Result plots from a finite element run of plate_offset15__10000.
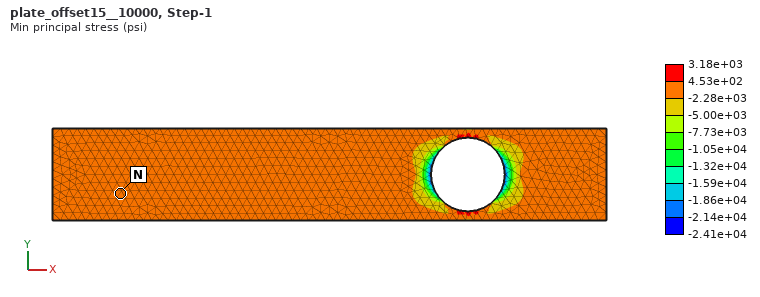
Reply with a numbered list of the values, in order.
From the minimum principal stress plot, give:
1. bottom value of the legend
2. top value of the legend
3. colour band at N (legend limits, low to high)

1. -2.41e+04 psi
2. 3.18e+03 psi
3. -2.28e+03 to 4.53e+02 psi
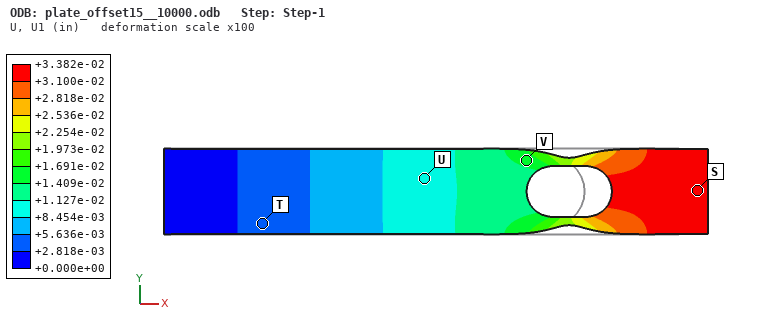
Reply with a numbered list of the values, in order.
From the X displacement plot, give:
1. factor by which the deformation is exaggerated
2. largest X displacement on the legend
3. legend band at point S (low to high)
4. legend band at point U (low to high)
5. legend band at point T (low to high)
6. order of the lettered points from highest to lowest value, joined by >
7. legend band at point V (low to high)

1. 100
2. +3.382e-02 in
3. +3.100e-02 to +3.382e-02 in
4. +8.454e-03 to +1.127e-02 in
5. +2.818e-03 to +5.636e-03 in
6. S > V > U > T
7. +1.409e-02 to +1.691e-02 in
